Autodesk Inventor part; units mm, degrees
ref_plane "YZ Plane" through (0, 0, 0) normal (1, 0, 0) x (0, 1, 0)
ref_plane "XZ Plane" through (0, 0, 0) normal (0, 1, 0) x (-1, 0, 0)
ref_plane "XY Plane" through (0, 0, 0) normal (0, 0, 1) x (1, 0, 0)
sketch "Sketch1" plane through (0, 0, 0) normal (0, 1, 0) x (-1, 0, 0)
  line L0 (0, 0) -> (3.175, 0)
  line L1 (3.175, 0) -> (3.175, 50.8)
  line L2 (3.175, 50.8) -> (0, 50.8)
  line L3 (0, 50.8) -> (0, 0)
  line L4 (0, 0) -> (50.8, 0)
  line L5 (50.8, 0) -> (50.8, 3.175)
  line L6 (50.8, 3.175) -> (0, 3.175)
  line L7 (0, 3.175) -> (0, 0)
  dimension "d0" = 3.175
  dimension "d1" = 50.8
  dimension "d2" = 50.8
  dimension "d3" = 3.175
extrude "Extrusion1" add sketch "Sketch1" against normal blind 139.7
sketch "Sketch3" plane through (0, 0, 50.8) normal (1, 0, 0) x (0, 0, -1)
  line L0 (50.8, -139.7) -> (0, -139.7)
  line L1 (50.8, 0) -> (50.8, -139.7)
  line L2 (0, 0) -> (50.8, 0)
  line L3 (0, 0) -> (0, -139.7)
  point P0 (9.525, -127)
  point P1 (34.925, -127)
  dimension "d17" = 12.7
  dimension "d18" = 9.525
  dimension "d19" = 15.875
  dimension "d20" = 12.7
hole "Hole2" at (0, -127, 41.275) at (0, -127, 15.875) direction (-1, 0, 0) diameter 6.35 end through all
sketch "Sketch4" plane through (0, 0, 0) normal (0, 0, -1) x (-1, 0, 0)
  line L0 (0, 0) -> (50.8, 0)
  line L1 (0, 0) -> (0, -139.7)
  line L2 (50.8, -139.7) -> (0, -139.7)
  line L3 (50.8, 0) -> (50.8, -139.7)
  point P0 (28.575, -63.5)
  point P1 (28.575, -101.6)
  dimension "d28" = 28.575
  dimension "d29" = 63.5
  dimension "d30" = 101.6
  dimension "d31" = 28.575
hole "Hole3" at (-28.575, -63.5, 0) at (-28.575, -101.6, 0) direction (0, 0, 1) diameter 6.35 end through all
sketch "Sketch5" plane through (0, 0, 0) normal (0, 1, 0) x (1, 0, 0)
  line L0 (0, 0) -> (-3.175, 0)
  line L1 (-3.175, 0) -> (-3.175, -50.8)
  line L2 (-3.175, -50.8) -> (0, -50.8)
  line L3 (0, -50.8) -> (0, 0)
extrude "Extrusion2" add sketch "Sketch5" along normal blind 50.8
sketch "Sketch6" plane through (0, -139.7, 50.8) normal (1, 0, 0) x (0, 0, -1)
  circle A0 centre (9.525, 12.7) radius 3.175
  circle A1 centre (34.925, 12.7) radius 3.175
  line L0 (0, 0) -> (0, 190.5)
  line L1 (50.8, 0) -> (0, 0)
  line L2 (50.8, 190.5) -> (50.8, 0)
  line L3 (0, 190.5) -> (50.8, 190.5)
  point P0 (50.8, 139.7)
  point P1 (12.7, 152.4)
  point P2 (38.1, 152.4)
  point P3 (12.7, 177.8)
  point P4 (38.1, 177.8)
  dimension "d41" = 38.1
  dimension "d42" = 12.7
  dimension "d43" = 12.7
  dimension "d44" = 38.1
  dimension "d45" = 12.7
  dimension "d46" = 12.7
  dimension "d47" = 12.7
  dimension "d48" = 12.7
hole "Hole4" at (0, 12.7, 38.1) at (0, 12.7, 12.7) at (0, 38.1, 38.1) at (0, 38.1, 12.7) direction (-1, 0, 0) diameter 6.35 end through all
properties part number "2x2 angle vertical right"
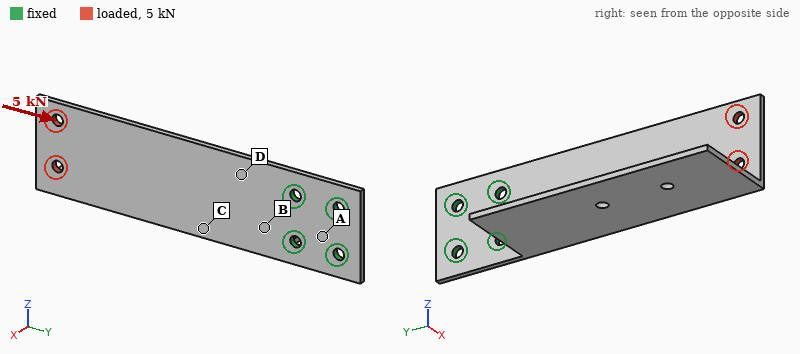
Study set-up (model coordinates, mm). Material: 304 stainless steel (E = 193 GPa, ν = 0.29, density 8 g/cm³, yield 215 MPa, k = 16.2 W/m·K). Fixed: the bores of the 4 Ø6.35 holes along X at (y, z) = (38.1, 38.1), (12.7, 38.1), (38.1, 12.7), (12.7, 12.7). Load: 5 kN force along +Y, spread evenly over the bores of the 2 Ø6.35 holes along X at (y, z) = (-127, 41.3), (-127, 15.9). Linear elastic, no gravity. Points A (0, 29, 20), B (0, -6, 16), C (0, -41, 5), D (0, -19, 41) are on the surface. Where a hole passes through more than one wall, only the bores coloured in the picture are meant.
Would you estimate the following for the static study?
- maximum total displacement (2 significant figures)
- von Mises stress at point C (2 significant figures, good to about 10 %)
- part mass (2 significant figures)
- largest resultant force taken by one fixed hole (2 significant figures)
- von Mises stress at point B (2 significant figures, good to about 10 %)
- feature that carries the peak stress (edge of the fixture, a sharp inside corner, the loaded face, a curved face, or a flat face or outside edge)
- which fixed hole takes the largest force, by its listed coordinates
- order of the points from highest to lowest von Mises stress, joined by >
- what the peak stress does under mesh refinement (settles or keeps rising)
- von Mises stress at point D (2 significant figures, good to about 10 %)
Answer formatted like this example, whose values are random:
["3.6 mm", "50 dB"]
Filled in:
["56 µm", "15 MPa", "410 g", "2.6 kN", "27 MPa", "edge of the fixture", "(12.7, 38.1)", "D > B > C > A", "keeps rising", "40 MPa"]
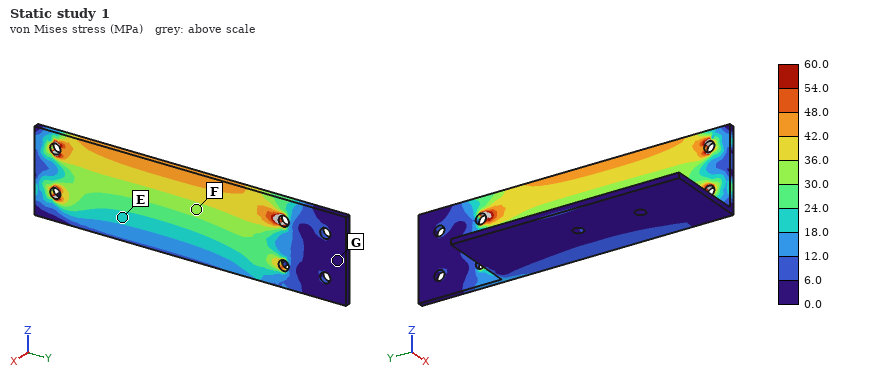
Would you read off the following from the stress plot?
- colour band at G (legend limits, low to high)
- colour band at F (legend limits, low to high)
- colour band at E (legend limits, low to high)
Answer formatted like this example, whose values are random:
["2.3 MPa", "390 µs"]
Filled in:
["0.0 to 6.0 MPa", "30.0 to 36.0 MPa", "18.0 to 24.0 MPa"]
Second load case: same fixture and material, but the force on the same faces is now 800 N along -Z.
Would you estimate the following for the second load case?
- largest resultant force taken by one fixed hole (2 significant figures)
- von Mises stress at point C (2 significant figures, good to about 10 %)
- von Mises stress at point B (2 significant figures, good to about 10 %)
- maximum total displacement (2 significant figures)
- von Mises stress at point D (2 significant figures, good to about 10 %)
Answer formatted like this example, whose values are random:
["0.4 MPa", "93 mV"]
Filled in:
["3.0 kN", "24 MPa", "35 MPa", "0.14 mm", "35 MPa"]
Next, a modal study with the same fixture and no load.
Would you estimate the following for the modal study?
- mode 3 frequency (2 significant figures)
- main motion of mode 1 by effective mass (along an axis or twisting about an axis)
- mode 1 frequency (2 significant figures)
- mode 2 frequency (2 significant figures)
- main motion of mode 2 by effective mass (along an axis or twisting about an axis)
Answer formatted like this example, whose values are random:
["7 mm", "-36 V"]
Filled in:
["960 Hz", "along X", "110 Hz", "330 Hz", "along Z"]
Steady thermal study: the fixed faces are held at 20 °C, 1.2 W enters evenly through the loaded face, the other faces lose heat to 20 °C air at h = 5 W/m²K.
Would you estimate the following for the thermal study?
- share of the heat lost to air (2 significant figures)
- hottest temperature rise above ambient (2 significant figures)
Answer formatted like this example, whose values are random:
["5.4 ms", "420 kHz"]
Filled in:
["83 %", "22 K"]
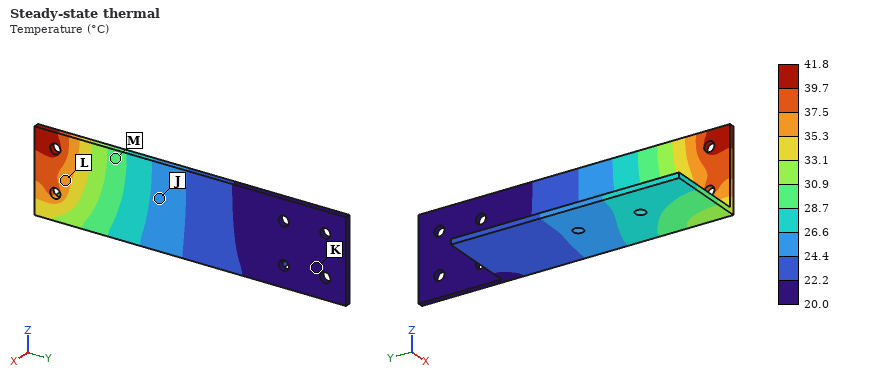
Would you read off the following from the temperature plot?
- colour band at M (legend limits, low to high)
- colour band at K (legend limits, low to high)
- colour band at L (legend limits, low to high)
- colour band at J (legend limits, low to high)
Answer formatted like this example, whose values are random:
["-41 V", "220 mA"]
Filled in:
["28.7 to 30.9 °C", "20.0 to 22.2 °C", "35.3 to 37.5 °C", "24.4 to 26.6 °C"]
